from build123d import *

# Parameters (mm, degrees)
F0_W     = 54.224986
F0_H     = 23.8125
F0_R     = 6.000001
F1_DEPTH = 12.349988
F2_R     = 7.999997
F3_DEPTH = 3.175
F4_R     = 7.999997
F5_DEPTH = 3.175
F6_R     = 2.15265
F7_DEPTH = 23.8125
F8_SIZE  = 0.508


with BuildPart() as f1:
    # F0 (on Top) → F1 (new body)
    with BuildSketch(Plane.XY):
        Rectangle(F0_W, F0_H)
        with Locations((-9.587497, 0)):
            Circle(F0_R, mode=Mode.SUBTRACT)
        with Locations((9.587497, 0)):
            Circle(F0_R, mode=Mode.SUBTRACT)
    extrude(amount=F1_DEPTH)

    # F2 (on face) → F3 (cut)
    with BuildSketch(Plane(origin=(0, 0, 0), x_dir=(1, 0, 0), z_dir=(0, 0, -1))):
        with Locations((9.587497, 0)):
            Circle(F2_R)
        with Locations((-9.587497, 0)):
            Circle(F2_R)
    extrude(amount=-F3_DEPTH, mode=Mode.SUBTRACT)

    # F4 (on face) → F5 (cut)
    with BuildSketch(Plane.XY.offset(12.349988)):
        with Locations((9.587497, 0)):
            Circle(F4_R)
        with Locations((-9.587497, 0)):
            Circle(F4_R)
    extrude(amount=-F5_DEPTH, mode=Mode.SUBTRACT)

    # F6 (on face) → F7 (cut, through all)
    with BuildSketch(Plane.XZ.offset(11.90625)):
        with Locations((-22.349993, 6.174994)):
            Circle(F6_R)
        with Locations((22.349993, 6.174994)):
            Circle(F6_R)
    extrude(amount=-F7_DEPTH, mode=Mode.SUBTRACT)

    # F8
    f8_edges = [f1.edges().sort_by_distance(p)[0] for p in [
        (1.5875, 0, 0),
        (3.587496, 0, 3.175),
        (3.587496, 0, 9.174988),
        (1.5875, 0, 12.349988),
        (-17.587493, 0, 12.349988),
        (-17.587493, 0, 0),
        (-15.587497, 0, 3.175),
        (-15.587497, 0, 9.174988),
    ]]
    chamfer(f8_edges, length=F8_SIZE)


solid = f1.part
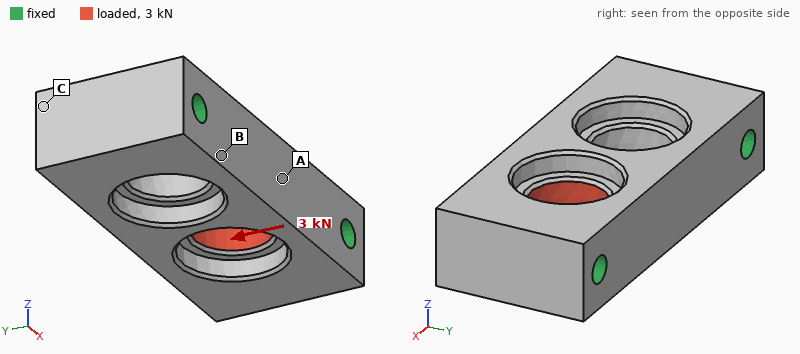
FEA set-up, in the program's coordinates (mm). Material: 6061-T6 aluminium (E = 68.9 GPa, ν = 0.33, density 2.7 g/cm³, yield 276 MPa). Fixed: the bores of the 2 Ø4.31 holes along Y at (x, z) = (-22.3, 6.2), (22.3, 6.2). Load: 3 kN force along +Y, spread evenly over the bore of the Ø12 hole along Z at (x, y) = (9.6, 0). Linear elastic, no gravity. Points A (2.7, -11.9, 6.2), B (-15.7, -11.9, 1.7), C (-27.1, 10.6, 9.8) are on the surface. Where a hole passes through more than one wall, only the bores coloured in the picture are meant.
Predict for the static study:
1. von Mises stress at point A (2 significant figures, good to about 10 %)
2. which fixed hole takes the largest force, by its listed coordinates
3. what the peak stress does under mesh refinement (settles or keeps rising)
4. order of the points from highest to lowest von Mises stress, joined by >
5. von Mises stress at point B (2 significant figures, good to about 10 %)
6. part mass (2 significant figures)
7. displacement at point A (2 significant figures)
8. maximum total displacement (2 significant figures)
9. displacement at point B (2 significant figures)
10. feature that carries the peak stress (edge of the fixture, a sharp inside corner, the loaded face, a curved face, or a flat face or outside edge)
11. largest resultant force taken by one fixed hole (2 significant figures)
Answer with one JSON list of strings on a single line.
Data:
["21 MPa", "(22.3, 6.2)", "keeps rising", "A > B > C", "17 MPa", "30 g", "11 µm", "12 µm", "2.1 µm", "edge of the fixture", "2.3 kN"]
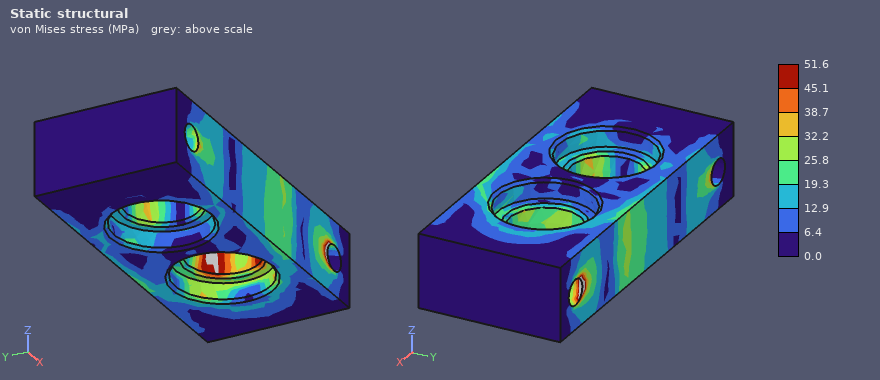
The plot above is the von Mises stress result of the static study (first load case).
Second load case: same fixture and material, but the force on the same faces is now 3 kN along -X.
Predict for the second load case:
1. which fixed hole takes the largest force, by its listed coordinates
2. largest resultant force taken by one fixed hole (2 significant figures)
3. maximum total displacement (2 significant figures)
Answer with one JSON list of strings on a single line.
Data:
["(22.3, 6.2)", "2.2 kN", "4.5 µm"]
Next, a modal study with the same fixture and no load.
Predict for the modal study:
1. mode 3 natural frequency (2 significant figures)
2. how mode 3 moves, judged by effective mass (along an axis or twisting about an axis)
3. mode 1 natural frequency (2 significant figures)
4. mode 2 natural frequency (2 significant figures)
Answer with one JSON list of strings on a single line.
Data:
["24 kHz", "twisting about X", "20 kHz", "20 kHz"]
